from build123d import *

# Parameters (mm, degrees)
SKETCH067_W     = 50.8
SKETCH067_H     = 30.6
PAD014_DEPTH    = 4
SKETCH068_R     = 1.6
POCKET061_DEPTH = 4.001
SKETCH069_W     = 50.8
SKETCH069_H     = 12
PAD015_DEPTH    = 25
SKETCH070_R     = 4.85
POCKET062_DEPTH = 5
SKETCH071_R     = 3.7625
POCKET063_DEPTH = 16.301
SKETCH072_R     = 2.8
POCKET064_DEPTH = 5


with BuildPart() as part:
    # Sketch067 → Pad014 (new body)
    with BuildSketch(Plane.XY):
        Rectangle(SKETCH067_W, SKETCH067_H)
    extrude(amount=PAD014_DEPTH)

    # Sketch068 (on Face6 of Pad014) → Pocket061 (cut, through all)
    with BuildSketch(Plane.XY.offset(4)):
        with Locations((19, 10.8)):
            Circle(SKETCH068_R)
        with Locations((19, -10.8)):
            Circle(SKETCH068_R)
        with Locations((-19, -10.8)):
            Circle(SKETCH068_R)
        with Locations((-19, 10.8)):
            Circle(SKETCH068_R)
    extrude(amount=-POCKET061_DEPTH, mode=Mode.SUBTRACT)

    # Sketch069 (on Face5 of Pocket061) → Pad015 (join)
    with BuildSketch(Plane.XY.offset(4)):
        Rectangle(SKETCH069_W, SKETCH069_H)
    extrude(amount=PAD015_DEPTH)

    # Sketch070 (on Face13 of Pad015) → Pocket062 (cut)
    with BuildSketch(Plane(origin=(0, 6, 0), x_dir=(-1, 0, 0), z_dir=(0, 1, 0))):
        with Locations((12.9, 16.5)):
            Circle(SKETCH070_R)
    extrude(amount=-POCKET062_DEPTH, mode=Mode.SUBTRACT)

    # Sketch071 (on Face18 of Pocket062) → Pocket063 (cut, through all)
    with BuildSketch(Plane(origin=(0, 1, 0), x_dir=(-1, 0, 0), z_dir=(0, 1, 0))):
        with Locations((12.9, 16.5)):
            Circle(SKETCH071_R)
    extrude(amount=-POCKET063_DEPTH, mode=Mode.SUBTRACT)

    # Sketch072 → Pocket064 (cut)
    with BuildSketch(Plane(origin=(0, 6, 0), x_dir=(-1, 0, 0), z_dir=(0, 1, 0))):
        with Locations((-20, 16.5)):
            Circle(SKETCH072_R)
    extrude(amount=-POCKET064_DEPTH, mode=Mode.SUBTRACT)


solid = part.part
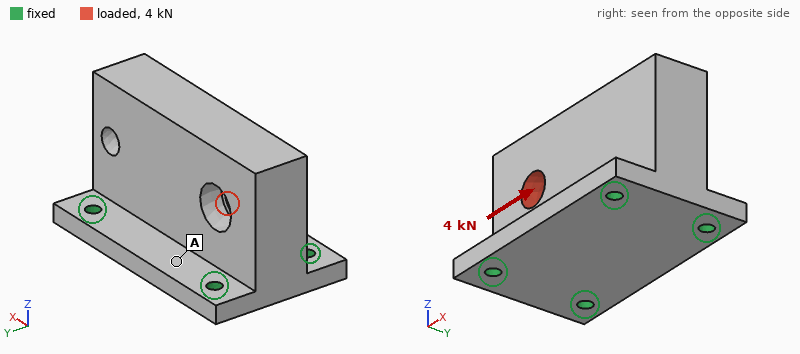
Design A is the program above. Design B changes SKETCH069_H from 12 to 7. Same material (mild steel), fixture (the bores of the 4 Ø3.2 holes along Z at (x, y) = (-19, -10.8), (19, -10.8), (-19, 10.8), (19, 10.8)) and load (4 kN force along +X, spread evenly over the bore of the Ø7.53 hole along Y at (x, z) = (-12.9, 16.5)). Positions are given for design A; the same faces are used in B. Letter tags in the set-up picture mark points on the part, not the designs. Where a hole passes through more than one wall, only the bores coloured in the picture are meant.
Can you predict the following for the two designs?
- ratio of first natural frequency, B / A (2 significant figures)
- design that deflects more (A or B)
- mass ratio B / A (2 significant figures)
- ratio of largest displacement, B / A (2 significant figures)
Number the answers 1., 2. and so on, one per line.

1. 0.81
2. B
3. 0.71
4. 1.6
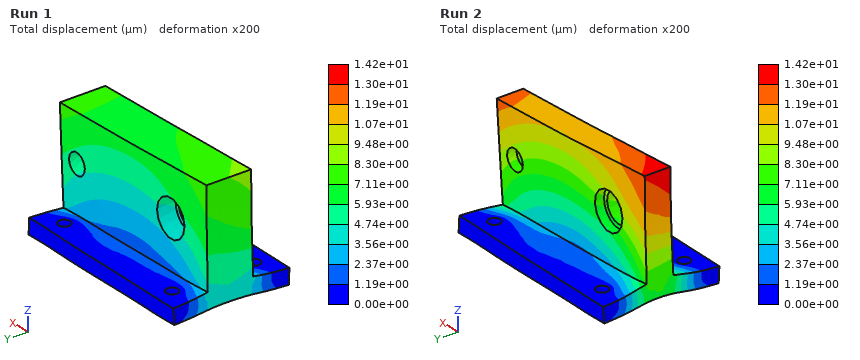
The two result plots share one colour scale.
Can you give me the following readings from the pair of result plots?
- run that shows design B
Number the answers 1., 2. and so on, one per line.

1. Run 2
